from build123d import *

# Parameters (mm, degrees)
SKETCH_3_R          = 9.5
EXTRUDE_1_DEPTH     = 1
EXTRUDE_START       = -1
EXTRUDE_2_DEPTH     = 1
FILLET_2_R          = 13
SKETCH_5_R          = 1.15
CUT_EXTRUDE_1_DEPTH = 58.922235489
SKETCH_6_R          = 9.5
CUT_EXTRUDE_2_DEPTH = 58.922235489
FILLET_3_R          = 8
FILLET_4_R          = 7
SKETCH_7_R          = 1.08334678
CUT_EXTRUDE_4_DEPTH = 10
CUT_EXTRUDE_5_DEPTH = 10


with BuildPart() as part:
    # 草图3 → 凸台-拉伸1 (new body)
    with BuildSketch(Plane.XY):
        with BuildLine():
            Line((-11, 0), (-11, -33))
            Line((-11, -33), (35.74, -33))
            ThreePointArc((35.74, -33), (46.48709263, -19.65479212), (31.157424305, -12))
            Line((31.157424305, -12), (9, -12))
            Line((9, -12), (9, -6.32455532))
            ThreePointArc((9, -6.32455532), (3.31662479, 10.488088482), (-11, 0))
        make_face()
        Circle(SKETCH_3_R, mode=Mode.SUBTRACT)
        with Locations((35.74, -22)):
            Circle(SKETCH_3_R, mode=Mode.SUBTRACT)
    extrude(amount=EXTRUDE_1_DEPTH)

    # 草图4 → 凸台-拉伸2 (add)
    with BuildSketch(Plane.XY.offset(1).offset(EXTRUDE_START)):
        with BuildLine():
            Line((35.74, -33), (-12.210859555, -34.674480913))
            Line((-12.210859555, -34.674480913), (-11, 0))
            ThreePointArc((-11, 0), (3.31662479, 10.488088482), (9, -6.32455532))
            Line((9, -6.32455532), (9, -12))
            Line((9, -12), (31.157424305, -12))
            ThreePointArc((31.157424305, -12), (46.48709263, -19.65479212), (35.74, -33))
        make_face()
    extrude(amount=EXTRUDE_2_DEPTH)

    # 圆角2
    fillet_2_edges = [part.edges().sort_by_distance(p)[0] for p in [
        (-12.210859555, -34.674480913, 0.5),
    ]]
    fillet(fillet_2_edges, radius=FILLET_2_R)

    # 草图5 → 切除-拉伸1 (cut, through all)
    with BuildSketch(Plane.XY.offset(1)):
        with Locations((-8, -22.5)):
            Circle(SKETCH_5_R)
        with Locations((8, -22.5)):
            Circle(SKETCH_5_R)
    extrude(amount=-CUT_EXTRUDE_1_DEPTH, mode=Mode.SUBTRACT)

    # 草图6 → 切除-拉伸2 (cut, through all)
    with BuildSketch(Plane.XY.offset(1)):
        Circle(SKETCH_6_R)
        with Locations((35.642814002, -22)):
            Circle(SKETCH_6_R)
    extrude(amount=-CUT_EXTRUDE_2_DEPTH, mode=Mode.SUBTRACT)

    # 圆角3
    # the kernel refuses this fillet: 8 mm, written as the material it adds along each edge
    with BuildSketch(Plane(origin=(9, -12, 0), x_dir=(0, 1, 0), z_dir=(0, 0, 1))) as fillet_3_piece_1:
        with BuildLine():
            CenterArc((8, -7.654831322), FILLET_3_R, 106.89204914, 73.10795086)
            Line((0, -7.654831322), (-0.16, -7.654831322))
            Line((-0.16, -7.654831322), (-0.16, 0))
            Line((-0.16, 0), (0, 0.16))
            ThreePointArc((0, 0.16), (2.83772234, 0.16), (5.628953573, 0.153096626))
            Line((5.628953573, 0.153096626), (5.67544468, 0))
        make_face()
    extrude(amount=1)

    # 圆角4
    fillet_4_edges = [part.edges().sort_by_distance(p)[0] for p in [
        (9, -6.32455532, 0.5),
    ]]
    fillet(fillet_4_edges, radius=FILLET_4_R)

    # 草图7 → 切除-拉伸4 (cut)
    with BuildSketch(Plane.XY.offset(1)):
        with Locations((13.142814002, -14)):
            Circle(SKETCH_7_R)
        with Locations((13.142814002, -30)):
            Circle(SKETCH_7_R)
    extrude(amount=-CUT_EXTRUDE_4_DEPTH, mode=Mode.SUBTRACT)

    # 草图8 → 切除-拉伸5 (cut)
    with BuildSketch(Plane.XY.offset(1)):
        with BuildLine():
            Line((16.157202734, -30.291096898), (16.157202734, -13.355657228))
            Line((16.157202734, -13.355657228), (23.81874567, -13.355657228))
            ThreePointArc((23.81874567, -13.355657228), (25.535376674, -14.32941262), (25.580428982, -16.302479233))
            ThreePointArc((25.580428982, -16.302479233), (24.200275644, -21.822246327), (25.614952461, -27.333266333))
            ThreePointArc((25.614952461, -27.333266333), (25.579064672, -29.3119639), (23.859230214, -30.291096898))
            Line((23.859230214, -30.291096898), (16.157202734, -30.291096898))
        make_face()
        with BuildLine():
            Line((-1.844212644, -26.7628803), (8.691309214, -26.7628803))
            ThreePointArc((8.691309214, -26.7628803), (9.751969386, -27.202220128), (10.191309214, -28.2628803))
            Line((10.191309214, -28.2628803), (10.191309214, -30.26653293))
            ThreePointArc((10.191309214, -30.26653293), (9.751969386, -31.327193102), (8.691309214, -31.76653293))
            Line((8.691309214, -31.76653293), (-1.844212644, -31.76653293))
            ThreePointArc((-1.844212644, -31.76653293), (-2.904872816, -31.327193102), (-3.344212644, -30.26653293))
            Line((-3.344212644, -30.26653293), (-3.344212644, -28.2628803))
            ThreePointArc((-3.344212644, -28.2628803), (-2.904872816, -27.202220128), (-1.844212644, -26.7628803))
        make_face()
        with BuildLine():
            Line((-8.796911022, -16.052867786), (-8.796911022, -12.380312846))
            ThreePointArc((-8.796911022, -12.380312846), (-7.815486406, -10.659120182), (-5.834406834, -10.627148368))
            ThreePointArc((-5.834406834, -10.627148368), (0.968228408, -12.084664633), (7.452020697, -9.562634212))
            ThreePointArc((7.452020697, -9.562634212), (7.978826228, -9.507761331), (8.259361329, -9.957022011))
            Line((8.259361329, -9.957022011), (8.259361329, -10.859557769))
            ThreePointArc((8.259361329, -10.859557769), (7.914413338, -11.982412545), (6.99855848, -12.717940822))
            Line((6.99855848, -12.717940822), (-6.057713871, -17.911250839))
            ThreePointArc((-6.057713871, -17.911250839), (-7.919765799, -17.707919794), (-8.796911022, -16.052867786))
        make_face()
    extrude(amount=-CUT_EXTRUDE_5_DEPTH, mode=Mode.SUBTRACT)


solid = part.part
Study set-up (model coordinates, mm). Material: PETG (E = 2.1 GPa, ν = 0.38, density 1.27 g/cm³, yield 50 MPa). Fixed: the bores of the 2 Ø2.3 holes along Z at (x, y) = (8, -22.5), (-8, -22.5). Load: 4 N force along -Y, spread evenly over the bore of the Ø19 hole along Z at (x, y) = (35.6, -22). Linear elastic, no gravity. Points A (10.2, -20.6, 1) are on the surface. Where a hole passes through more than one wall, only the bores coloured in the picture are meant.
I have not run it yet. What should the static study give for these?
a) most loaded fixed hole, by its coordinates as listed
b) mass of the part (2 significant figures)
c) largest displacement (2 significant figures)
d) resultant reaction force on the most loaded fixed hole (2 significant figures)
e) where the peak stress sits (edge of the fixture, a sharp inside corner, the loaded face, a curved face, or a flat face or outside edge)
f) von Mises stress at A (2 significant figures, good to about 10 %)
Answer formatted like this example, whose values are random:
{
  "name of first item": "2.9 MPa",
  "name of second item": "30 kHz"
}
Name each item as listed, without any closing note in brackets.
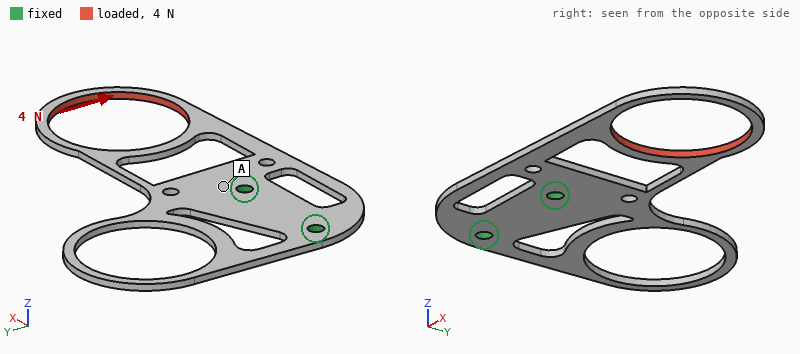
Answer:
{
  "most loaded fixed hole, by its coordinates as listed": "(8, -22.5)",
  "mass of the part": "0.99 g",
  "largest displacement": "0.83 mm",
  "resultant reaction force on the most loaded fixed hole": "9.6 N",
  "where the peak stress sits": "a curved face",
  "von Mises stress at A": "1.7 MPa"
}
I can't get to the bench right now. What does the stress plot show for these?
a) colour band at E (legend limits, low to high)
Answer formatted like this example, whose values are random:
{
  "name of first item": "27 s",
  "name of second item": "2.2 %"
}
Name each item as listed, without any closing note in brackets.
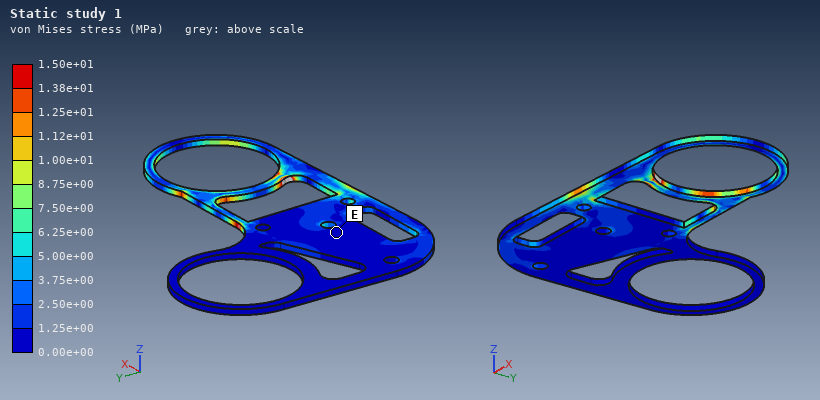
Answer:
{
  "colour band at E": "0.00e+00 to 1.25e+00 MPa"
}
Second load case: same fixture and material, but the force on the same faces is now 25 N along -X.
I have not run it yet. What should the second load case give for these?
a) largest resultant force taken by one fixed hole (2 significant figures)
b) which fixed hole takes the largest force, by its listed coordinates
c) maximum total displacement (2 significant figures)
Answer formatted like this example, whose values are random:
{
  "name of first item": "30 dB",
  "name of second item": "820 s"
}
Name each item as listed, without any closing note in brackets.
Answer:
{
  "largest resultant force taken by one fixed hole": "17 N",
  "which fixed hole takes the largest force, by its listed coordinates": "(8, -22.5)",
  "maximum total displacement": "0.37 mm"
}
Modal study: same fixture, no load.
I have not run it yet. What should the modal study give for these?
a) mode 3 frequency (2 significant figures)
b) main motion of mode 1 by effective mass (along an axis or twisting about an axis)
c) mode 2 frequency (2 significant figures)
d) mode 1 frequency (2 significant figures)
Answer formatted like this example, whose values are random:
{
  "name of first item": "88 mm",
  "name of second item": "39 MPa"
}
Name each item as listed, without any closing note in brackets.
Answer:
{
  "mode 3 frequency": "430 Hz",
  "main motion of mode 1 by effective mass": "along Z",
  "mode 2 frequency": "270 Hz",
  "mode 1 frequency": "160 Hz"
}
